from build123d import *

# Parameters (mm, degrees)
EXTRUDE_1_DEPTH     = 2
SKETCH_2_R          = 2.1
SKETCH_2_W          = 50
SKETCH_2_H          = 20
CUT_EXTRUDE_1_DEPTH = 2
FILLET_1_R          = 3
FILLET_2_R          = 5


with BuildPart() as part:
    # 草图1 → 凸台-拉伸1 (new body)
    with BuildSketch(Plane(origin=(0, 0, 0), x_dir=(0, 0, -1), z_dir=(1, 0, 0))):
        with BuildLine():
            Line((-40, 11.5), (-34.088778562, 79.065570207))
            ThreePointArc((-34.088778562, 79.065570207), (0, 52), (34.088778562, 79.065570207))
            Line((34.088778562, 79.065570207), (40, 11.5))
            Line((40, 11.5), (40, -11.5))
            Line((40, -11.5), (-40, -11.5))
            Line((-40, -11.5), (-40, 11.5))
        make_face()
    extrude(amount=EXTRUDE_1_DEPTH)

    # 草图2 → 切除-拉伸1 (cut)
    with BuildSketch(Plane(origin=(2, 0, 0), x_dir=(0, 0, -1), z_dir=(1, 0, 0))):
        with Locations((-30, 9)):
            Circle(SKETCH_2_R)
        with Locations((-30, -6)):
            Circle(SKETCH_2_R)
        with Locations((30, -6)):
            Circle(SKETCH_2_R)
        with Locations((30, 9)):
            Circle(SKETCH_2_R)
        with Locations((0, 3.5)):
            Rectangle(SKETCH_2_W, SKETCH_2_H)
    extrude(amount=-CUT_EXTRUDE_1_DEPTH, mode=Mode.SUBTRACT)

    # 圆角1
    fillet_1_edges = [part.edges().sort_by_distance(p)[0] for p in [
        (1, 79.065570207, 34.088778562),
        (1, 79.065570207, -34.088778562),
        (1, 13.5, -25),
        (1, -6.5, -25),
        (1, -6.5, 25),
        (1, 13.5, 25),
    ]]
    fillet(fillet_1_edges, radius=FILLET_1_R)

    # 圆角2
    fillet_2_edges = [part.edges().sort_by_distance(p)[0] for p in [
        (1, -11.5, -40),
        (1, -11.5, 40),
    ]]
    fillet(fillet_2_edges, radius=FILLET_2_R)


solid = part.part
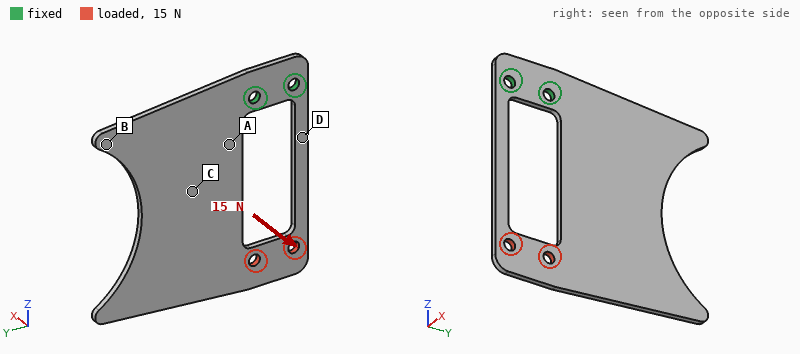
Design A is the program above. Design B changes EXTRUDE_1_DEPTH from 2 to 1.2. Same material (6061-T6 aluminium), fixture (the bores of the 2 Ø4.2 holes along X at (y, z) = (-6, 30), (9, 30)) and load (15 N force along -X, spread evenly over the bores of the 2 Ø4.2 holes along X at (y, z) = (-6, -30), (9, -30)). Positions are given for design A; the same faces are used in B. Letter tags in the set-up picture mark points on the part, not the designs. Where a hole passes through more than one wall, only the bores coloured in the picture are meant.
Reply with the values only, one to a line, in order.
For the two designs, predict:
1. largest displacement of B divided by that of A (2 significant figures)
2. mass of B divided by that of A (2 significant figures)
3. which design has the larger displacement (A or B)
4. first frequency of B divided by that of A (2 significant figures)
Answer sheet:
4.5
0.60
B
0.61
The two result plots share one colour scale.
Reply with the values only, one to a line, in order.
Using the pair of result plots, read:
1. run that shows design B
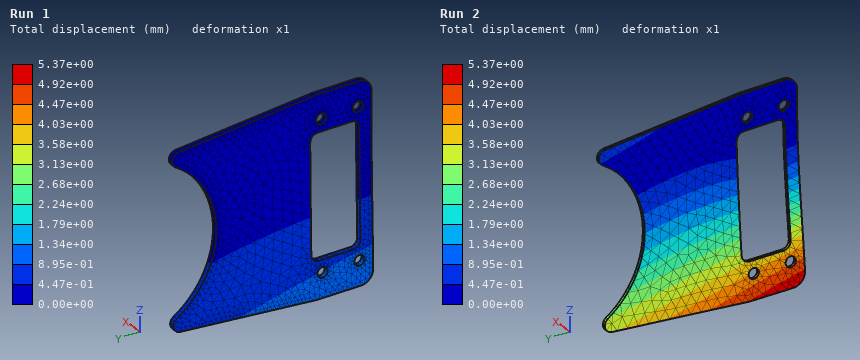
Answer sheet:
Run 2
